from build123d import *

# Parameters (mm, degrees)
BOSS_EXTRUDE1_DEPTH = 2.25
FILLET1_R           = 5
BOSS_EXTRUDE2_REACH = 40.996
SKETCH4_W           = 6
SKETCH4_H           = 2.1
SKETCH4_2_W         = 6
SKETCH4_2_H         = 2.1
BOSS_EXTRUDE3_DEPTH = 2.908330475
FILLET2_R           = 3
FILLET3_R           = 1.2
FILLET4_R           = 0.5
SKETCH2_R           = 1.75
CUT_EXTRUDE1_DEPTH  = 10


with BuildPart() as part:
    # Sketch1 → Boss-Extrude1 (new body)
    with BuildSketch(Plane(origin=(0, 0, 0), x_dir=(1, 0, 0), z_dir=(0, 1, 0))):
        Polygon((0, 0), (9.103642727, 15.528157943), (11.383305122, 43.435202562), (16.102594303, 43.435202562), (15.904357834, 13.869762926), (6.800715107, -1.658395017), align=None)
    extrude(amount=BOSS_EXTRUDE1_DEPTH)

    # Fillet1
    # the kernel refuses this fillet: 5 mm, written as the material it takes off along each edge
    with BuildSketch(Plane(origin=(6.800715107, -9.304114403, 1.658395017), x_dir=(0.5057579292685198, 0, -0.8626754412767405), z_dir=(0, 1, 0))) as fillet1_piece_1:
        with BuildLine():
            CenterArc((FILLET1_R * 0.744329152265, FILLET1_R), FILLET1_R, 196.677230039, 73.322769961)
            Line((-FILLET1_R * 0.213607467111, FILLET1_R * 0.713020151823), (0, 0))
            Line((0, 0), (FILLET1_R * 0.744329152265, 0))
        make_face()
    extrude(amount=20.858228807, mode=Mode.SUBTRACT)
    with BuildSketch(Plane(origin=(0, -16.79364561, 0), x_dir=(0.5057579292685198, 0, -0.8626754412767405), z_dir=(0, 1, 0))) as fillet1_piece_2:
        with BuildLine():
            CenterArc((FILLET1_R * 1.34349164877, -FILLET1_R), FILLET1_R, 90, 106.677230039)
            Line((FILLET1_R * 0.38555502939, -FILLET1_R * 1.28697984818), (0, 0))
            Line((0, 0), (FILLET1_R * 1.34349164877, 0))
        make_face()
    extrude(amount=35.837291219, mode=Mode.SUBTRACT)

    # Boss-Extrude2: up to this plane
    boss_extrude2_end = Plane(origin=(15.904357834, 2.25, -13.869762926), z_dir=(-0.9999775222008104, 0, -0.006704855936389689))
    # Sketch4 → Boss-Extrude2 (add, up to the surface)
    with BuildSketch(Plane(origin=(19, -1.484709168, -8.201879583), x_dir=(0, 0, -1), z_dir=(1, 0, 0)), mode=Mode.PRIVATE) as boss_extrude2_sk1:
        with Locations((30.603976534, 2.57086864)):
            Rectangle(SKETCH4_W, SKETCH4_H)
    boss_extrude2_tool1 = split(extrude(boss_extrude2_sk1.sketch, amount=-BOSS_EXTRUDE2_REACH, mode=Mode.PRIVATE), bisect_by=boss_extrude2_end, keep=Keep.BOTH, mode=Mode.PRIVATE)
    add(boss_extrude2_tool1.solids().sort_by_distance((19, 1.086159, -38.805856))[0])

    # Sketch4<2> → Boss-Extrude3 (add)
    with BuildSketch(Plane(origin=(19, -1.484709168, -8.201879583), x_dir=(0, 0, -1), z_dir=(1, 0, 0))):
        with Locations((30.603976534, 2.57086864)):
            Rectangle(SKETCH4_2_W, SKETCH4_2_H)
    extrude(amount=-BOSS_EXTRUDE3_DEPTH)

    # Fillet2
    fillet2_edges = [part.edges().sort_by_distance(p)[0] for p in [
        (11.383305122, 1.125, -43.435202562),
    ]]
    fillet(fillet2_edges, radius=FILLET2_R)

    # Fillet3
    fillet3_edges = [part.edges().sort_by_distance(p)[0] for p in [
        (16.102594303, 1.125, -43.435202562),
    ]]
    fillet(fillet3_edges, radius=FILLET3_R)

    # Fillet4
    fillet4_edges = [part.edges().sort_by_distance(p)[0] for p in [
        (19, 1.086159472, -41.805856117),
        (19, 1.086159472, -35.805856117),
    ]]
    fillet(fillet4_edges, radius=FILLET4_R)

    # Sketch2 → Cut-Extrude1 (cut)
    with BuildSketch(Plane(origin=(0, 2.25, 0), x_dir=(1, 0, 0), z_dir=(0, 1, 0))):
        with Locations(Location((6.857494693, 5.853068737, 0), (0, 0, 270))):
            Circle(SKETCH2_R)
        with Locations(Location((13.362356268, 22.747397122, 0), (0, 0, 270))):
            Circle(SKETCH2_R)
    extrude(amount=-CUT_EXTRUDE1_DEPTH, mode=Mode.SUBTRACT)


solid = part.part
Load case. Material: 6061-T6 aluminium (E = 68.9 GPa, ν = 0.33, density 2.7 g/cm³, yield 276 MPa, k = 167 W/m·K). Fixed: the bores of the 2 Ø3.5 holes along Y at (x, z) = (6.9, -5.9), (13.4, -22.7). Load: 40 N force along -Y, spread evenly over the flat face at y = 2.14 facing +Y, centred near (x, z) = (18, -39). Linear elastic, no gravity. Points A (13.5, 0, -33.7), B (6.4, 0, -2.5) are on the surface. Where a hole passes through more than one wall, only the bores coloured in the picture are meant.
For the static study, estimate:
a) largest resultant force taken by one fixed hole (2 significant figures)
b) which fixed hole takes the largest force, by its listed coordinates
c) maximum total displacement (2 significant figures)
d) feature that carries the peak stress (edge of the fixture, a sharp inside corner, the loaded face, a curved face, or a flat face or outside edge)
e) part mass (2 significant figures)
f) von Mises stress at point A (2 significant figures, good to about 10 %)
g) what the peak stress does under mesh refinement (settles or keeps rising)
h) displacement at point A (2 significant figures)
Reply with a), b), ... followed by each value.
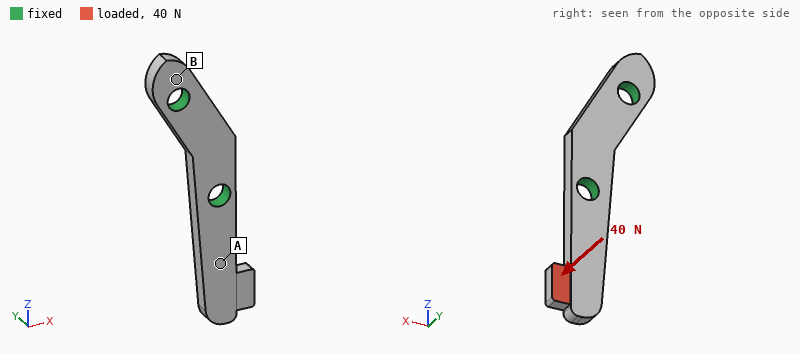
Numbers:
a) 40 N
b) (13.4, -22.7)
c) 0.18 mm
d) edge of the fixture
e) 1.6 g
f) 59 MPa
g) keeps rising
h) 0.058 mm
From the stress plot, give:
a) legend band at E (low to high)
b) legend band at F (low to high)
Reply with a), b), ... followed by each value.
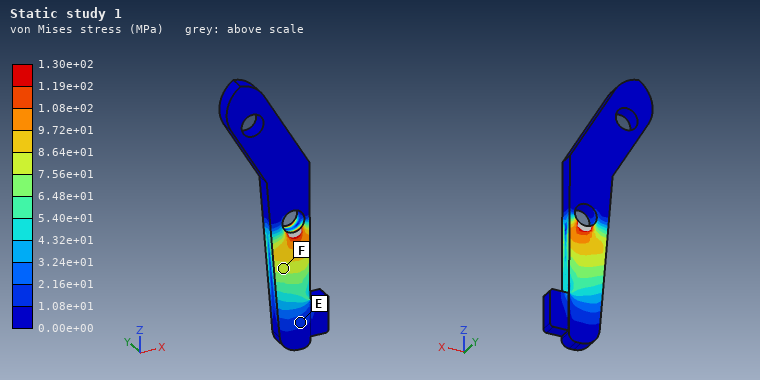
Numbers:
a) 1.08e+01 to 2.16e+01 MPa
b) 7.56e+01 to 8.64e+01 MPa
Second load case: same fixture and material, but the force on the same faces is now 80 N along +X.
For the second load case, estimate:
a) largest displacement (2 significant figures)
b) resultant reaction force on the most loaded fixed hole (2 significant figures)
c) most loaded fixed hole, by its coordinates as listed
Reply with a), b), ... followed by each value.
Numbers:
a) 66 µm
b) 88 N
c) (13.4, -22.7)
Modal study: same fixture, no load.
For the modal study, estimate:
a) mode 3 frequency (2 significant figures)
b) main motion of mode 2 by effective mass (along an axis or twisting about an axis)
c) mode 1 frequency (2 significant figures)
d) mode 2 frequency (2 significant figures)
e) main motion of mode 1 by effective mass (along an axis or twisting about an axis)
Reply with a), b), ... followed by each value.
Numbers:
a) 20 kHz
b) along X
c) 4700 Hz
d) 10 kHz
e) along Y
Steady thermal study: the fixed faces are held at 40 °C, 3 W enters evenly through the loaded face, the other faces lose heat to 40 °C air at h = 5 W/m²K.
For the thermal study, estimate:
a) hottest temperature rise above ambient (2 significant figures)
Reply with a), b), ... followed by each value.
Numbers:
a) 24 K
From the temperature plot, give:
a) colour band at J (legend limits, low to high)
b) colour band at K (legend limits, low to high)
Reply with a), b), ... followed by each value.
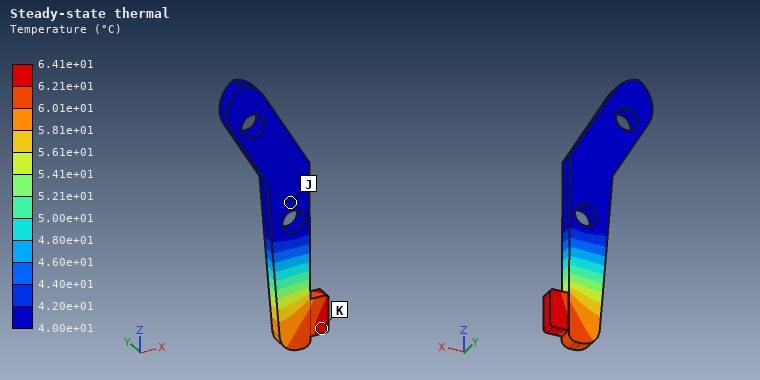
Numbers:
a) 4.00e+01 to 4.20e+01 °C
b) 6.21e+01 to 6.41e+01 °C
